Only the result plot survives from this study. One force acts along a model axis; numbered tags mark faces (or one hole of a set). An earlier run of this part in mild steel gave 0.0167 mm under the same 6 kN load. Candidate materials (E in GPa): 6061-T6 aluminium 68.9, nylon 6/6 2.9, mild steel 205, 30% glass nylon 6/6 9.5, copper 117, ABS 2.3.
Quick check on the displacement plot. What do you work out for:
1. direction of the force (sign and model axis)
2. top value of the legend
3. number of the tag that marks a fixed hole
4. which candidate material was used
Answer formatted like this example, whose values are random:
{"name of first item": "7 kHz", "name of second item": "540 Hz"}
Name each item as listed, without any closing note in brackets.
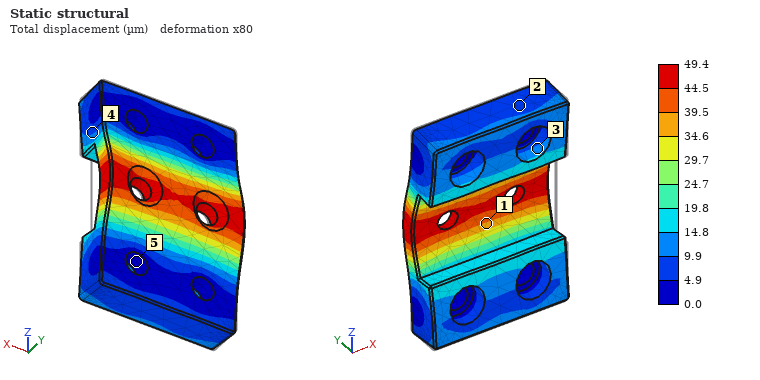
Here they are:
{"direction of the force": "+Y", "top value of the legend": "49.4 µm", "number of the tag that marks a fixed hole": "5", "which candidate material was used": "6061-T6 aluminium"}
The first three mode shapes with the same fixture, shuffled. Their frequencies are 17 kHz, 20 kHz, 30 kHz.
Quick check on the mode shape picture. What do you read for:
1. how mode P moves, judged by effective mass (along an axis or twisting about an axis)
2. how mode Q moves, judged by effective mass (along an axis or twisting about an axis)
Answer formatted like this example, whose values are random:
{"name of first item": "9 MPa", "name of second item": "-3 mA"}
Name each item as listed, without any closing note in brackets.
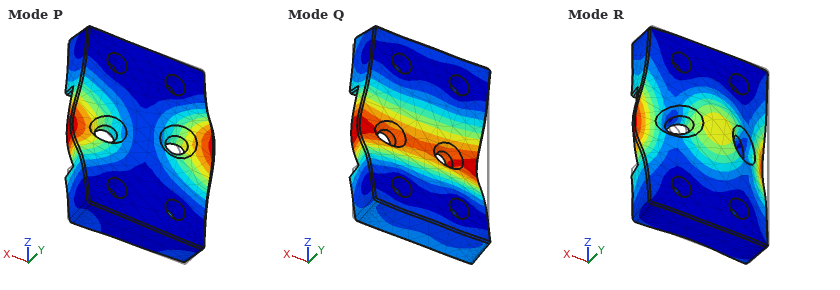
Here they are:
{"how mode P moves, judged by effective mass": "twisting about Z", "how mode Q moves, judged by effective mass": "along Y"}
